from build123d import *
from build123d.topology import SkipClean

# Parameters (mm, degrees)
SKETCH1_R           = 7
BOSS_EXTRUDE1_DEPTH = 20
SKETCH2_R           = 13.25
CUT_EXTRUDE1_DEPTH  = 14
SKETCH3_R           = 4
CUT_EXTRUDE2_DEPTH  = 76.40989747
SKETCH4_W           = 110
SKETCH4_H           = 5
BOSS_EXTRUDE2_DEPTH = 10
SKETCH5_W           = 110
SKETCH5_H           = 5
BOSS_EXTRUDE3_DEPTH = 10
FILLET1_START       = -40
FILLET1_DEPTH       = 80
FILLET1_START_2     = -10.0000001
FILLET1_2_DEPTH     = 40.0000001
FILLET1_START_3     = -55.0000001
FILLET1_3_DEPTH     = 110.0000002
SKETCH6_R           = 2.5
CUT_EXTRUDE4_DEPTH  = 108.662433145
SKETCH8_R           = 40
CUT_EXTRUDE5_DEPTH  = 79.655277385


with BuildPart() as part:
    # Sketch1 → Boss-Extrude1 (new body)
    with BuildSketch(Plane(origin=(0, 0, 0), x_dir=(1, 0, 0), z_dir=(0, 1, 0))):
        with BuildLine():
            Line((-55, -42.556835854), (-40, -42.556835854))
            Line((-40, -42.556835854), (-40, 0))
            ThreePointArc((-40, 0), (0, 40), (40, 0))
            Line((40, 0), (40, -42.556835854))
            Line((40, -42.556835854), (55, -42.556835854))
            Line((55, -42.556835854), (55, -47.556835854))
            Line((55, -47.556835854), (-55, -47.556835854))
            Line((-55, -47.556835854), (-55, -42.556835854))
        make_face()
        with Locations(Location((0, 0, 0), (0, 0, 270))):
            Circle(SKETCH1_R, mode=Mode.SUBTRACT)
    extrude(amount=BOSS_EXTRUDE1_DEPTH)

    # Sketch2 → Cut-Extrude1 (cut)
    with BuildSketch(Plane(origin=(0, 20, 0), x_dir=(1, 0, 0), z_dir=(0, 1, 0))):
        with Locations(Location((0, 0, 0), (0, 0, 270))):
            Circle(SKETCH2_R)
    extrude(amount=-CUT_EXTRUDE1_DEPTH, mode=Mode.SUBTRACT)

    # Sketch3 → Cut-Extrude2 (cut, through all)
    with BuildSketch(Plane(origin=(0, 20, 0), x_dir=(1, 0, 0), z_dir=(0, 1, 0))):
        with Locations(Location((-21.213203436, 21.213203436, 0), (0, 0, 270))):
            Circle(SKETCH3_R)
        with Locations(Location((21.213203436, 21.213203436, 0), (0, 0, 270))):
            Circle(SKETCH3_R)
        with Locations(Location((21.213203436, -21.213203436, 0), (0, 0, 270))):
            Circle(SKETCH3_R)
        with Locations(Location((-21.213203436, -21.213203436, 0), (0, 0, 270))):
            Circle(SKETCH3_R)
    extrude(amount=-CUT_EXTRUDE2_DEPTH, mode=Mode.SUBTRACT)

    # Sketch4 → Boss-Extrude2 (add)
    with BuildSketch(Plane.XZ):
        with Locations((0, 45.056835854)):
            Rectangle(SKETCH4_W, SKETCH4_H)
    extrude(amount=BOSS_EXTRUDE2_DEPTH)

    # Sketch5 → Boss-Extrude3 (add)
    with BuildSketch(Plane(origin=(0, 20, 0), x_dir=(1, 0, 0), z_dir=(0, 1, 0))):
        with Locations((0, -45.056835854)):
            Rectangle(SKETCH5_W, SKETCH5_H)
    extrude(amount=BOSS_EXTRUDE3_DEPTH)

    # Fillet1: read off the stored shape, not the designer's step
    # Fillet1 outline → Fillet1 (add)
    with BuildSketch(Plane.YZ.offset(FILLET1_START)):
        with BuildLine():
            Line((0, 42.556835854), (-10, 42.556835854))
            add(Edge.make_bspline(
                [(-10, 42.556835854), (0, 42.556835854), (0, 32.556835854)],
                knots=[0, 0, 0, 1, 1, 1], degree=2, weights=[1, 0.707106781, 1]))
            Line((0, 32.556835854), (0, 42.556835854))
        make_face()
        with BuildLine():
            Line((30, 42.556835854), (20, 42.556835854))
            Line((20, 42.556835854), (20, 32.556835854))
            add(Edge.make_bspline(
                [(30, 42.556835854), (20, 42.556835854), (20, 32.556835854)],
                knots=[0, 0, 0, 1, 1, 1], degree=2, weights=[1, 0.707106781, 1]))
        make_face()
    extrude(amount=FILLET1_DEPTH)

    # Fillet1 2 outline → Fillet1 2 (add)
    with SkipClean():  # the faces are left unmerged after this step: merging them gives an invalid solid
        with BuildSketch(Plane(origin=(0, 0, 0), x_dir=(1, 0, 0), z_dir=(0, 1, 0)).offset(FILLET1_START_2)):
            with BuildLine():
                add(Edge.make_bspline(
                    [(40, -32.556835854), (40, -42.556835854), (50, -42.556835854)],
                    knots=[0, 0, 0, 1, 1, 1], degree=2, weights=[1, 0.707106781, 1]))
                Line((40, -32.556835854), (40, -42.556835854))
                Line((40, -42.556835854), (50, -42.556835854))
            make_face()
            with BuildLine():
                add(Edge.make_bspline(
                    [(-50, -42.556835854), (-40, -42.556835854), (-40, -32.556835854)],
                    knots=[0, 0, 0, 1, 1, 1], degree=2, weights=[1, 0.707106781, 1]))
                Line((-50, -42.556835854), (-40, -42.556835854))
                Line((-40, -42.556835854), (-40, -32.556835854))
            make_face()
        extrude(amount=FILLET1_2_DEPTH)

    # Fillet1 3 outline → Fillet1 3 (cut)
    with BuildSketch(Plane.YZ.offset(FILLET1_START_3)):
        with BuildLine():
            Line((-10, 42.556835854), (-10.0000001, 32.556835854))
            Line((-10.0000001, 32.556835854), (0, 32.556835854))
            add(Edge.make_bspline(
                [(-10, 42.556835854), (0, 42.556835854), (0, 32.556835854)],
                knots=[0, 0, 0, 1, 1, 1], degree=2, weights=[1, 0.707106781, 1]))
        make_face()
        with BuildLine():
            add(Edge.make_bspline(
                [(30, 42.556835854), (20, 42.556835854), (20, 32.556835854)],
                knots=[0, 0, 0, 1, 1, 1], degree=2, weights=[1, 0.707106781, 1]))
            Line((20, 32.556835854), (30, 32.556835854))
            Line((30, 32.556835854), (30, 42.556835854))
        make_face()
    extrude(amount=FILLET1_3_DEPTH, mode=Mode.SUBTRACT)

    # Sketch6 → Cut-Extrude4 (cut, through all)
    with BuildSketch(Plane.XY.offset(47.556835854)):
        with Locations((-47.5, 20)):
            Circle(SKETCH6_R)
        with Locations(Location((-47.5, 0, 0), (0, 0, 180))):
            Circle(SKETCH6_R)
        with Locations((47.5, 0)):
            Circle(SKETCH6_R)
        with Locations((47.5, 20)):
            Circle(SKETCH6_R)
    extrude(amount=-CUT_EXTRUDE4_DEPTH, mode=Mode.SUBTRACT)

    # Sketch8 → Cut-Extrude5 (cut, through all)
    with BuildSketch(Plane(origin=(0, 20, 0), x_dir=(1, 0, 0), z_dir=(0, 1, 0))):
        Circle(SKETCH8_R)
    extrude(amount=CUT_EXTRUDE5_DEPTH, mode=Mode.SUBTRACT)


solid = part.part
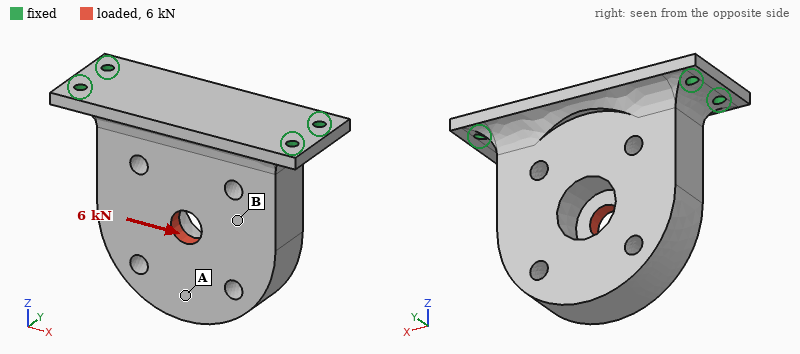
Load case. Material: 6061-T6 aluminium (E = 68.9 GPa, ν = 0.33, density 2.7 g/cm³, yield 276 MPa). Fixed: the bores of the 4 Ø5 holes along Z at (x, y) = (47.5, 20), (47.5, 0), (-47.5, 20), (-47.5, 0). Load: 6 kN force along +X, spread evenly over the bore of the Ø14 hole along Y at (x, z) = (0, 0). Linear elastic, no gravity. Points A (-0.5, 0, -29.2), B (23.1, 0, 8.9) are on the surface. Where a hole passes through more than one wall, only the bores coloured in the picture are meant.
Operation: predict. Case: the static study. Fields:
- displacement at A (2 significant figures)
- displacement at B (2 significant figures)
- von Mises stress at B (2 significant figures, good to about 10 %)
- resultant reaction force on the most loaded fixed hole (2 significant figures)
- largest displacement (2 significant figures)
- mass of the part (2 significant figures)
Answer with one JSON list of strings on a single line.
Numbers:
["32 µm", "19 µm", "17 MPa", "2.4 kN", "34 µm", "360 g"]
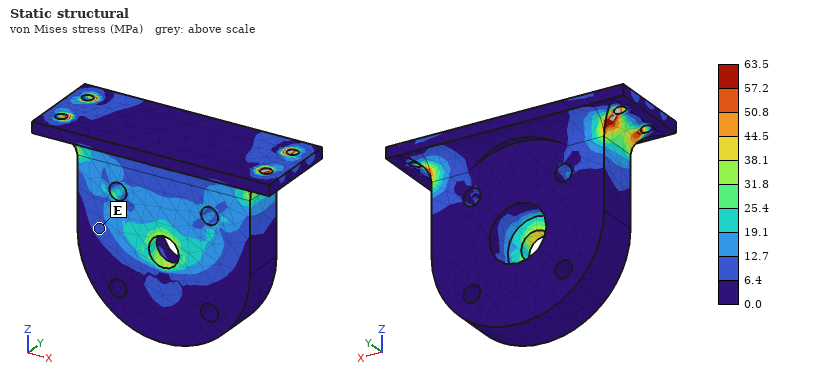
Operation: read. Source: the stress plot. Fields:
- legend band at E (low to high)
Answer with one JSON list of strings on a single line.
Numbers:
["6.4 to 12.7 MPa"]
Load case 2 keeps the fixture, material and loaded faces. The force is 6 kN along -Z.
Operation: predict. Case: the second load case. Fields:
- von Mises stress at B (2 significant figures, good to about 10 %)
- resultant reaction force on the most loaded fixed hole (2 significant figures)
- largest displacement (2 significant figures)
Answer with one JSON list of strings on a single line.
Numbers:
["11 MPa", "2.7 kN", "96 µm"]
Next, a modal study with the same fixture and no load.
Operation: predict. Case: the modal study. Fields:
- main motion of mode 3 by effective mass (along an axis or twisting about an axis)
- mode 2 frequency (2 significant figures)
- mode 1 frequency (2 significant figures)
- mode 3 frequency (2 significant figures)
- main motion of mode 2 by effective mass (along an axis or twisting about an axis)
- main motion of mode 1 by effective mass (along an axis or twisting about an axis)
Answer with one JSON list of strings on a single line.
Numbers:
["twisting about Z", "5000 Hz", "1400 Hz", "5400 Hz", "along X", "along Y"]
